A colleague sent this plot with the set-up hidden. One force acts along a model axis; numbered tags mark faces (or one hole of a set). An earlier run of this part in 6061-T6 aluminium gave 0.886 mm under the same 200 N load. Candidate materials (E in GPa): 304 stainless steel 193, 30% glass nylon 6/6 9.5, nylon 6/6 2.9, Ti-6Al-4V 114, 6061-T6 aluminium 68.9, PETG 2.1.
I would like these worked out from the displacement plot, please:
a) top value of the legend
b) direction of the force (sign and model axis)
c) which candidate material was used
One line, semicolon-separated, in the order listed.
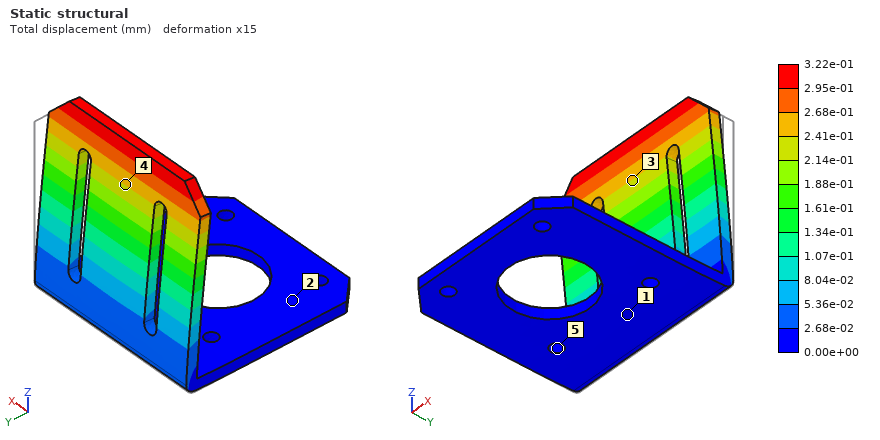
3.22e-01 mm; -Y; 304 stainless steel
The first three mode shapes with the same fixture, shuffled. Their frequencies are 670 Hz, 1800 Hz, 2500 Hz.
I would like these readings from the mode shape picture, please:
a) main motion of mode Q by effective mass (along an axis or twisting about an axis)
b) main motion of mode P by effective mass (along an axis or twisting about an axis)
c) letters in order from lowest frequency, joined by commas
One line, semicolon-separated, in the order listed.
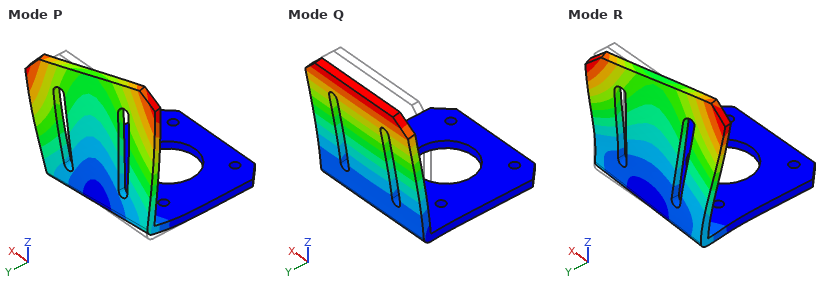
along Y; along X; Q, P, R
